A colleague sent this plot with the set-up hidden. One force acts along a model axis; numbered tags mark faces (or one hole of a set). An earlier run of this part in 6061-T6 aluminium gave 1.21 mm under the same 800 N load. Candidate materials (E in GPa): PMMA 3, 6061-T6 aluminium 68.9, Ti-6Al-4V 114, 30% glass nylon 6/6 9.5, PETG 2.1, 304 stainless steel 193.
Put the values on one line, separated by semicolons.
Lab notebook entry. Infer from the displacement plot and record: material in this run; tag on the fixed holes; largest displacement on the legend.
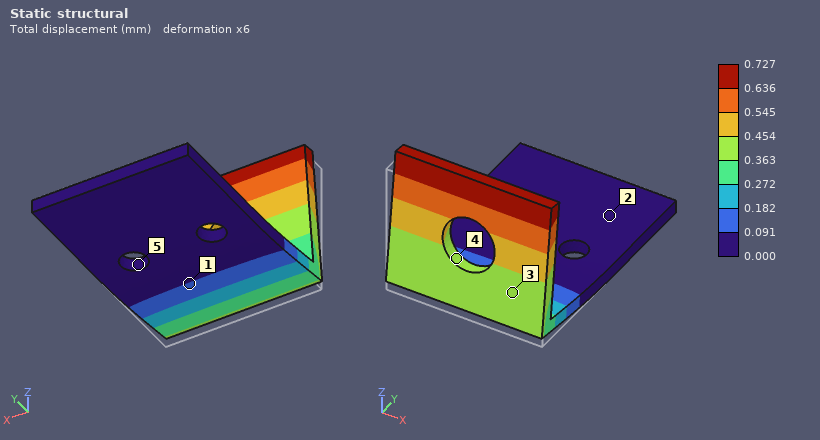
Ti-6Al-4V; 5; 0.727 mm
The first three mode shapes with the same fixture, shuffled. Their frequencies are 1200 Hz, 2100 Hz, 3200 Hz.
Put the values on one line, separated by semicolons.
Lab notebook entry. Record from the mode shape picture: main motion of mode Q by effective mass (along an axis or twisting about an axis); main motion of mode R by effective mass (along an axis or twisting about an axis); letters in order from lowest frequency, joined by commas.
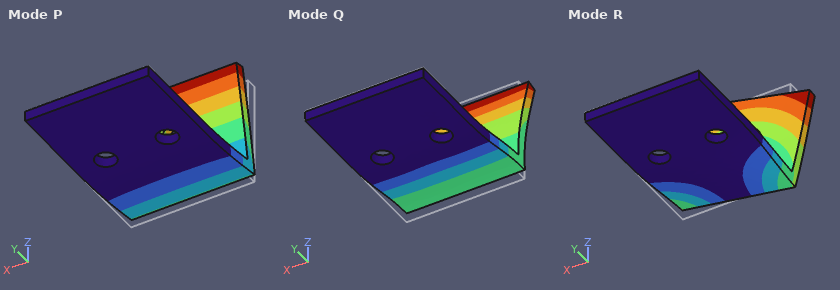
along Z; along X; P, R, Q
